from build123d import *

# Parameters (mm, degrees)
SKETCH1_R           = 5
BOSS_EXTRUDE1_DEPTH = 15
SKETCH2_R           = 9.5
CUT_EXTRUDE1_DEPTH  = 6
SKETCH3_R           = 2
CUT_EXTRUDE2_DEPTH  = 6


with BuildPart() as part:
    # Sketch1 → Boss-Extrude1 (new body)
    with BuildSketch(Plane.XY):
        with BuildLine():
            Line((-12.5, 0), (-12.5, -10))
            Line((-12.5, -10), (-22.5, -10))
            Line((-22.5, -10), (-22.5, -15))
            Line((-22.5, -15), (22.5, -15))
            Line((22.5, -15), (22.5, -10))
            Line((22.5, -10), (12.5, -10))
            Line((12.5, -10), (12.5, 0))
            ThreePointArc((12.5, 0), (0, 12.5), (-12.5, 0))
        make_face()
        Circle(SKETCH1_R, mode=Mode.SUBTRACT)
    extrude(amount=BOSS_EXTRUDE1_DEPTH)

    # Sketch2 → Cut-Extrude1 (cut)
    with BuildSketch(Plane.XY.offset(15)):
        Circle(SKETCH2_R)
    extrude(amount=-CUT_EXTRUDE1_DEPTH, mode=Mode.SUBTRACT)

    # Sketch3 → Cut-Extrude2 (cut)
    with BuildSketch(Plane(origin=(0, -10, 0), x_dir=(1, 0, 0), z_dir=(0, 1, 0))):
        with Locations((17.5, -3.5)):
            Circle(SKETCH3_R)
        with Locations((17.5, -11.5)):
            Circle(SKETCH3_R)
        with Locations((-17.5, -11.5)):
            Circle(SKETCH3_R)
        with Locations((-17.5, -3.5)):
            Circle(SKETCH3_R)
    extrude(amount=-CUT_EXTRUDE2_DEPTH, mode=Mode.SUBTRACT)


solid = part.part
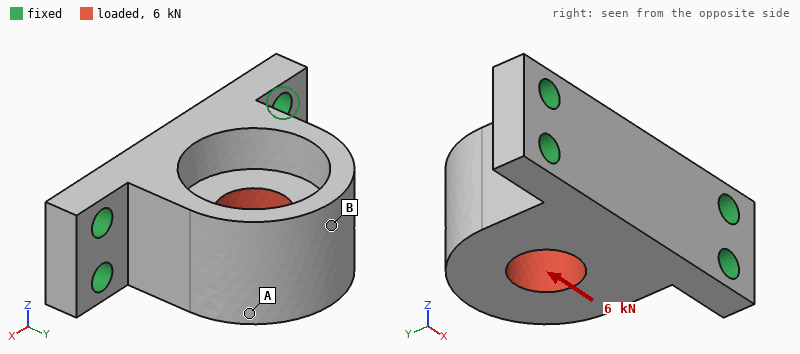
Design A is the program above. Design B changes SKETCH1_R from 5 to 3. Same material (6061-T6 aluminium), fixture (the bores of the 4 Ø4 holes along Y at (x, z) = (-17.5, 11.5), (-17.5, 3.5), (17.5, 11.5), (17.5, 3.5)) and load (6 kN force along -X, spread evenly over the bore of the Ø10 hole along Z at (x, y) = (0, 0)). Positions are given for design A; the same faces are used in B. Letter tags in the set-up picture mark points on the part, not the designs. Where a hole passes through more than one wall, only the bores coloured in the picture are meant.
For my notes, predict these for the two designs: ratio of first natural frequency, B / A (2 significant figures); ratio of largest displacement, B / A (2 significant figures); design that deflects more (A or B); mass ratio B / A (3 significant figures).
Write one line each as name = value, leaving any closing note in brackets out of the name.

ratio of first natural frequency, B / A = 0.97
ratio of largest displacement, B / A = 0.82
design that deflects more = A
mass ratio B / A = 1.06
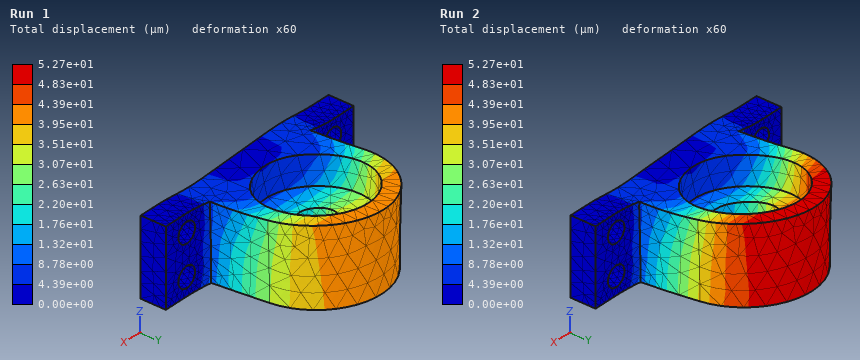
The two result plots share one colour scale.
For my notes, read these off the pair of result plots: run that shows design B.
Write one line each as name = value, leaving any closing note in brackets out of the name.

run that shows design B = Run 1
